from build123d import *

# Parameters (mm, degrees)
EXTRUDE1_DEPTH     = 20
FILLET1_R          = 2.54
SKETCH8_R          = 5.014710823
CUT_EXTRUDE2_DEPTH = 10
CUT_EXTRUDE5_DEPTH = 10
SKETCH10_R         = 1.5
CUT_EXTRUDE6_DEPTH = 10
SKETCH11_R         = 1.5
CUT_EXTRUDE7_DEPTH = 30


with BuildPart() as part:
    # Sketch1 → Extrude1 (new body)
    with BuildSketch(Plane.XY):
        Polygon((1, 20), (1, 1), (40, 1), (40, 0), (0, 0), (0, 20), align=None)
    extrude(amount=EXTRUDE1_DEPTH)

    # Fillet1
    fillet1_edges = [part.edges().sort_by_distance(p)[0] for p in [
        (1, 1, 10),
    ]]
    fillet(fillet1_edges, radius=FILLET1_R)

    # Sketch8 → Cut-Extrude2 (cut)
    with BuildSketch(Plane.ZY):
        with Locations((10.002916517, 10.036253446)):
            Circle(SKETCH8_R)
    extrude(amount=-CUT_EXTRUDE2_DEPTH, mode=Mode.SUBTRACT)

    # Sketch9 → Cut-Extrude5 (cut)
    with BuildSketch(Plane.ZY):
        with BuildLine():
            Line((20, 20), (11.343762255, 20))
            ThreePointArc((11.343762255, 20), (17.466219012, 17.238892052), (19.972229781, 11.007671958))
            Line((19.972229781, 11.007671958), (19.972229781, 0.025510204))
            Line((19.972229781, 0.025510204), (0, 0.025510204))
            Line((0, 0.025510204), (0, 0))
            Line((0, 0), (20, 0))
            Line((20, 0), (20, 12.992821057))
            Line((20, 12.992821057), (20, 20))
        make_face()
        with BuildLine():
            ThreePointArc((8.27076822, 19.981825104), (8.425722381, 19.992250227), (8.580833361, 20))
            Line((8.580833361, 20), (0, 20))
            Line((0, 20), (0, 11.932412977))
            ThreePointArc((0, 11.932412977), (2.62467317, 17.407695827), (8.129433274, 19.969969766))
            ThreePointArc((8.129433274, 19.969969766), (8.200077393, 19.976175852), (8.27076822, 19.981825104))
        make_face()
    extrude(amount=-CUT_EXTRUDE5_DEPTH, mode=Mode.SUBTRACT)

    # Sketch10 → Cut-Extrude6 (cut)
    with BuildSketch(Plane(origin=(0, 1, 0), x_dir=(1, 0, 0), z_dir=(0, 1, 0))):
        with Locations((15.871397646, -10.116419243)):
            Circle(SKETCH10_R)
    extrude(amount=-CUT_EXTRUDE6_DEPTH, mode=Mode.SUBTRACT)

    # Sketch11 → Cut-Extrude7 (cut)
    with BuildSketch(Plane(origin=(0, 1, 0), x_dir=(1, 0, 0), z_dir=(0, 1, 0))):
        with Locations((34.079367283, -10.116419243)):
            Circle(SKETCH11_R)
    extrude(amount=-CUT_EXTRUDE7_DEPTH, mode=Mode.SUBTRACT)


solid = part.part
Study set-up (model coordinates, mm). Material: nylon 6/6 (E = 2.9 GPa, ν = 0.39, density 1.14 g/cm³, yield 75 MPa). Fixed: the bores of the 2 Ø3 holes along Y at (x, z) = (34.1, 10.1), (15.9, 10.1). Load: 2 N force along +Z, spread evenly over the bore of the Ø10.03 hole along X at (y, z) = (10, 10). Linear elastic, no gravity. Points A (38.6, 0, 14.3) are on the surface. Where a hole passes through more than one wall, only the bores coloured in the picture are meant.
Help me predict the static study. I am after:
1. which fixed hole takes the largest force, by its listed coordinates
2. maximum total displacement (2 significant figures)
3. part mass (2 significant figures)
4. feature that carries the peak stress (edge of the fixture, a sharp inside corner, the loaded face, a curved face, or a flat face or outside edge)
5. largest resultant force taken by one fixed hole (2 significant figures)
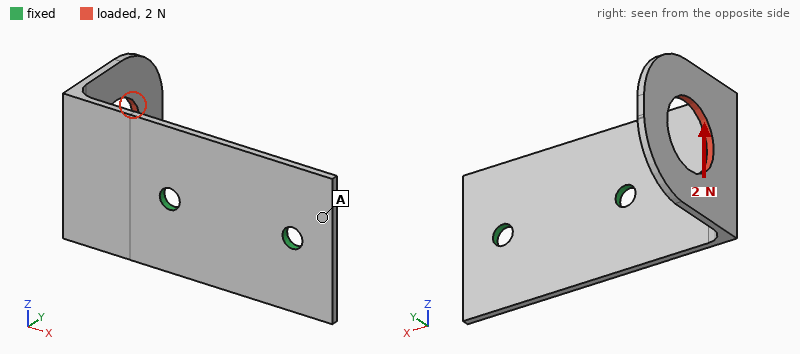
(15.9, 10.1)
0.57 mm
1.2 g
a flat face or outside edge
3.3 N
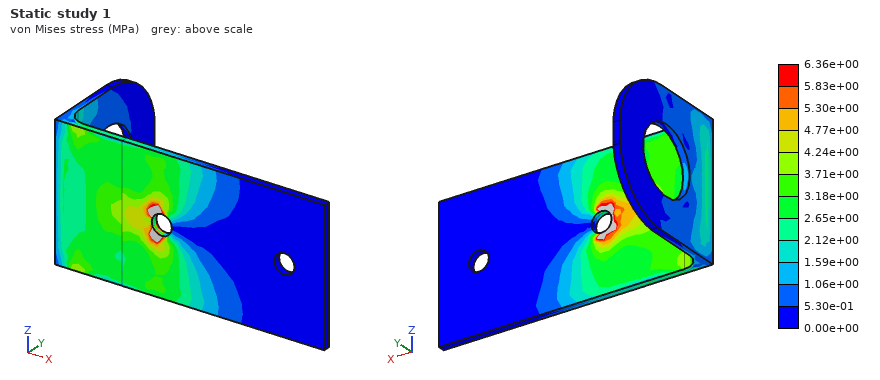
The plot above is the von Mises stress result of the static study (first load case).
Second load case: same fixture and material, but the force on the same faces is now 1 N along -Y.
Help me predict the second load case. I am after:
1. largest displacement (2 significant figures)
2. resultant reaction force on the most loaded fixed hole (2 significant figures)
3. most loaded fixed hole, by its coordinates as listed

0.50 mm
1.2 N
(15.9, 10.1)
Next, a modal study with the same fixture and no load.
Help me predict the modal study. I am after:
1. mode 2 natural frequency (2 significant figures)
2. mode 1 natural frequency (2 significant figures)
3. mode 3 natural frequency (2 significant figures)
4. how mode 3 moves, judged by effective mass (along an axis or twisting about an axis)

560 Hz
360 Hz
950 Hz
along Y
